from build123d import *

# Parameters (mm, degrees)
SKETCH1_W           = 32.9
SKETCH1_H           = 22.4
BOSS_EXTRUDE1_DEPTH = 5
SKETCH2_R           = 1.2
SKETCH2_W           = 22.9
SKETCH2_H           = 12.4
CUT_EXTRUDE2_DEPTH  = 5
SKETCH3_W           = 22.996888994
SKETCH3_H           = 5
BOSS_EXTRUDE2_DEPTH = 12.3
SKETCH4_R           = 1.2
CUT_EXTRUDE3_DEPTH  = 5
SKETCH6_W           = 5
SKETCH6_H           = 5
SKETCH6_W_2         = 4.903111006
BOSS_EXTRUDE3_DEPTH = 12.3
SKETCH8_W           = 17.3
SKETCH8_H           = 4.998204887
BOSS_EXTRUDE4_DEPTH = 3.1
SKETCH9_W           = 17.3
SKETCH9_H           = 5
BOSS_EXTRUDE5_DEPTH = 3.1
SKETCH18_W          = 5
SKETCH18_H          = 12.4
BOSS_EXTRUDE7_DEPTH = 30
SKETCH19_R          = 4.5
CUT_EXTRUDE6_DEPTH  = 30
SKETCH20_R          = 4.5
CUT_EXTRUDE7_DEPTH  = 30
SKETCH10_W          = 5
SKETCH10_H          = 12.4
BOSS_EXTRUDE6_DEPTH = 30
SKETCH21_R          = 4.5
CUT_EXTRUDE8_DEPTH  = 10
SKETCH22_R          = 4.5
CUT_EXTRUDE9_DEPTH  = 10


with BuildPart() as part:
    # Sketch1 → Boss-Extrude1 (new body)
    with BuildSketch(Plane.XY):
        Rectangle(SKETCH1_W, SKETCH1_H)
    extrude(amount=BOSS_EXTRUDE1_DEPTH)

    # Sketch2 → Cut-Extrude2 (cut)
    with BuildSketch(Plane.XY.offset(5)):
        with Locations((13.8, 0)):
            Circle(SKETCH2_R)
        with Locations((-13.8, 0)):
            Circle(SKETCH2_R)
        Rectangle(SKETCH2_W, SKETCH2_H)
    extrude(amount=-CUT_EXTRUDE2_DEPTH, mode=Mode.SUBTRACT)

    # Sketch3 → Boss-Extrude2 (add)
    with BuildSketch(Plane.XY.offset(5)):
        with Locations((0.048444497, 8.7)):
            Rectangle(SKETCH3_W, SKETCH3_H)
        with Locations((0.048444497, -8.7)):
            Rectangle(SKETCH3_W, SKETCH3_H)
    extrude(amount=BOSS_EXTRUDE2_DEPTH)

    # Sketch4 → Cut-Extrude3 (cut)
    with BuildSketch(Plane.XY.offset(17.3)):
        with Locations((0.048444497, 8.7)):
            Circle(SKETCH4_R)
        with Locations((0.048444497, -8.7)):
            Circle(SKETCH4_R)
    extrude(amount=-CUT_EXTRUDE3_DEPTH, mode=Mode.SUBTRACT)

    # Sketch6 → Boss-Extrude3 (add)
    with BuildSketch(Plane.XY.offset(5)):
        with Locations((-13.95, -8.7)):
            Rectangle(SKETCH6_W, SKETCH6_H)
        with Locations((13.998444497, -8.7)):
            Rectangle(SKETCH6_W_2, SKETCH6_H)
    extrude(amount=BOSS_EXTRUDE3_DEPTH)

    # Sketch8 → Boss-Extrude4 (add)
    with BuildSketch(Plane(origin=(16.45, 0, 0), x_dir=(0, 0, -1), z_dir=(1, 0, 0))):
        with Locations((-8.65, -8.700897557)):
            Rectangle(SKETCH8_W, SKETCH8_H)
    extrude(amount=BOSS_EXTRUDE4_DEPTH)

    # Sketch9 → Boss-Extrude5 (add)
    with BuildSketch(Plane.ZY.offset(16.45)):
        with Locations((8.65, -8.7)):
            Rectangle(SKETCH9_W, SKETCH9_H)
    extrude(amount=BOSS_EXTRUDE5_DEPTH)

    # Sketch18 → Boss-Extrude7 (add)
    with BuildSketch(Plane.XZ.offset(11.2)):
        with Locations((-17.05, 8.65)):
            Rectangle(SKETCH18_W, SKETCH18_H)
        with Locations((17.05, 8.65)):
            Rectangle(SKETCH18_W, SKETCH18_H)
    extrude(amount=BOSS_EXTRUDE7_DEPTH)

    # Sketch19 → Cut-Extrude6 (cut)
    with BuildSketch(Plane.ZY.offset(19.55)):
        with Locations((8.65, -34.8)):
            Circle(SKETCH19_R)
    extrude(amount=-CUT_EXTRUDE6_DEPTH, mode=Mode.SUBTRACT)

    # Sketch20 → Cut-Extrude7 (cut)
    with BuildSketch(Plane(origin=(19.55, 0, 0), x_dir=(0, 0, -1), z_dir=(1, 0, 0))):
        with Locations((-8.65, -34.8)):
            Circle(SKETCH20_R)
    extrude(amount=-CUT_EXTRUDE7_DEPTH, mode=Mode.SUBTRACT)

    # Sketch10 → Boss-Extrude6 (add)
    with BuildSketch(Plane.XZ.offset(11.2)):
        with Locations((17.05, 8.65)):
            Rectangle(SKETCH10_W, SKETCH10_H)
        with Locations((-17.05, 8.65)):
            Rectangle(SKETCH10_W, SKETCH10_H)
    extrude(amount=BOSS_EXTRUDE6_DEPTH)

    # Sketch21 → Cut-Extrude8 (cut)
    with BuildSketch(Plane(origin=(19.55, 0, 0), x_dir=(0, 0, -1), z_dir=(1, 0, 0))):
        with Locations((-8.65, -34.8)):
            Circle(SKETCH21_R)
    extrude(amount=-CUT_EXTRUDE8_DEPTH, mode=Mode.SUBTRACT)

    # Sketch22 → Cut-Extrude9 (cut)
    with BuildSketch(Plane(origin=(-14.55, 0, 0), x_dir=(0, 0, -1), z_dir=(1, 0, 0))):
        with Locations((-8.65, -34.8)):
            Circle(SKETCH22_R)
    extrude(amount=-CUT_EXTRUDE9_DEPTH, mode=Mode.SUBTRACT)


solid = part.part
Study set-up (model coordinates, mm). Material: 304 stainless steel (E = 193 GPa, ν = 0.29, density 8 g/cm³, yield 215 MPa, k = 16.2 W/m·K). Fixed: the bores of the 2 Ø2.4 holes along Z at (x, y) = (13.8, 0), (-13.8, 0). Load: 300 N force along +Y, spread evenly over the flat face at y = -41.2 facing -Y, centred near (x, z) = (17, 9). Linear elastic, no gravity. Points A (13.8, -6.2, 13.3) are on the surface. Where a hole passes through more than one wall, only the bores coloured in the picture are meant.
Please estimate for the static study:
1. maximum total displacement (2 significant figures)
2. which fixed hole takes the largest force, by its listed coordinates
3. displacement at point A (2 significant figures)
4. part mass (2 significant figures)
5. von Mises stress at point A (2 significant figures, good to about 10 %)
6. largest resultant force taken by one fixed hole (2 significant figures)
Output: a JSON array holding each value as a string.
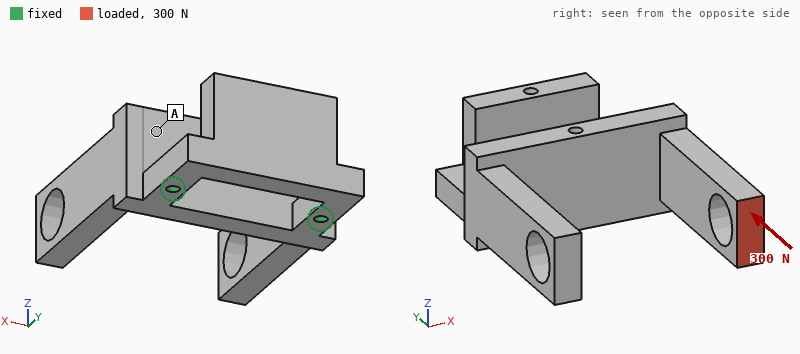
["38 µm", "(13.8, 0)", "10 µm", "74 g", "6.7 MPa", "330 N"]
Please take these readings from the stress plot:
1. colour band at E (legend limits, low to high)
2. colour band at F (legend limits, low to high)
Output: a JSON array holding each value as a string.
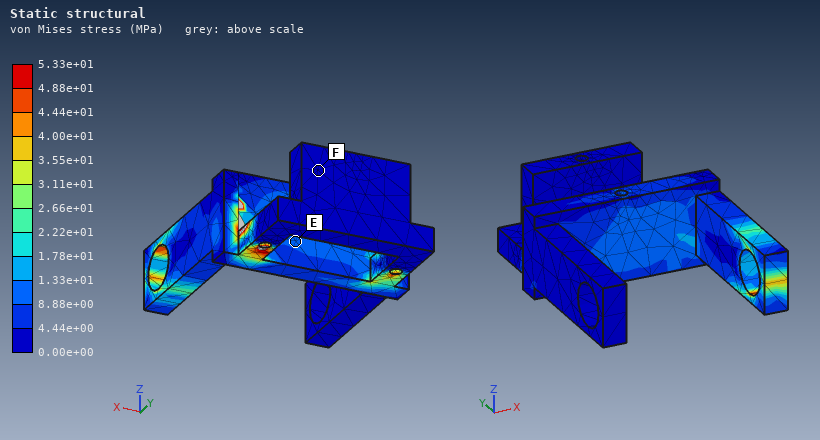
["8.88e+00 to 1.33e+01 MPa", "0.00e+00 to 4.44e+00 MPa"]
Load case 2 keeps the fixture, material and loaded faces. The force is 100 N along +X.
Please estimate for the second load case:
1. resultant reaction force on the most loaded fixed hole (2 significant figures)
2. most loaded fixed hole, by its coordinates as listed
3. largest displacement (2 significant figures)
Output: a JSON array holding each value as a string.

["220 N", "(-13.8, 0)", "72 µm"]
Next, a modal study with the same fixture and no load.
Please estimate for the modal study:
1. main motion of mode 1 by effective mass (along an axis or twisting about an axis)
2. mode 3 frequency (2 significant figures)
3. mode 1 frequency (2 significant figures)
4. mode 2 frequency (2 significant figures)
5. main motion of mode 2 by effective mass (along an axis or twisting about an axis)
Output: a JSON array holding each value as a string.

["along Z", "3600 Hz", "2000 Hz", "3200 Hz", "along X"]
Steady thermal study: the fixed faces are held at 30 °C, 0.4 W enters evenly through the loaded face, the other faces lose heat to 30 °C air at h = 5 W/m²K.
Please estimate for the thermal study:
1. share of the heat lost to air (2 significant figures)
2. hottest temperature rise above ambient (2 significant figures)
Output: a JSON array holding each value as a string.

["24 %", "23 K"]
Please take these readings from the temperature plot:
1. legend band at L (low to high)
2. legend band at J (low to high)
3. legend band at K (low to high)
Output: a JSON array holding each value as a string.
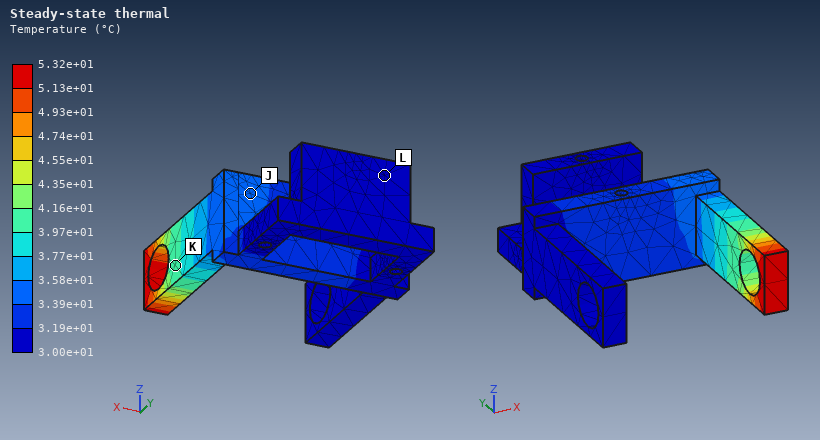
["3.00e+01 to 3.19e+01 °C", "3.39e+01 to 3.58e+01 °C", "3.97e+01 to 4.16e+01 °C"]
